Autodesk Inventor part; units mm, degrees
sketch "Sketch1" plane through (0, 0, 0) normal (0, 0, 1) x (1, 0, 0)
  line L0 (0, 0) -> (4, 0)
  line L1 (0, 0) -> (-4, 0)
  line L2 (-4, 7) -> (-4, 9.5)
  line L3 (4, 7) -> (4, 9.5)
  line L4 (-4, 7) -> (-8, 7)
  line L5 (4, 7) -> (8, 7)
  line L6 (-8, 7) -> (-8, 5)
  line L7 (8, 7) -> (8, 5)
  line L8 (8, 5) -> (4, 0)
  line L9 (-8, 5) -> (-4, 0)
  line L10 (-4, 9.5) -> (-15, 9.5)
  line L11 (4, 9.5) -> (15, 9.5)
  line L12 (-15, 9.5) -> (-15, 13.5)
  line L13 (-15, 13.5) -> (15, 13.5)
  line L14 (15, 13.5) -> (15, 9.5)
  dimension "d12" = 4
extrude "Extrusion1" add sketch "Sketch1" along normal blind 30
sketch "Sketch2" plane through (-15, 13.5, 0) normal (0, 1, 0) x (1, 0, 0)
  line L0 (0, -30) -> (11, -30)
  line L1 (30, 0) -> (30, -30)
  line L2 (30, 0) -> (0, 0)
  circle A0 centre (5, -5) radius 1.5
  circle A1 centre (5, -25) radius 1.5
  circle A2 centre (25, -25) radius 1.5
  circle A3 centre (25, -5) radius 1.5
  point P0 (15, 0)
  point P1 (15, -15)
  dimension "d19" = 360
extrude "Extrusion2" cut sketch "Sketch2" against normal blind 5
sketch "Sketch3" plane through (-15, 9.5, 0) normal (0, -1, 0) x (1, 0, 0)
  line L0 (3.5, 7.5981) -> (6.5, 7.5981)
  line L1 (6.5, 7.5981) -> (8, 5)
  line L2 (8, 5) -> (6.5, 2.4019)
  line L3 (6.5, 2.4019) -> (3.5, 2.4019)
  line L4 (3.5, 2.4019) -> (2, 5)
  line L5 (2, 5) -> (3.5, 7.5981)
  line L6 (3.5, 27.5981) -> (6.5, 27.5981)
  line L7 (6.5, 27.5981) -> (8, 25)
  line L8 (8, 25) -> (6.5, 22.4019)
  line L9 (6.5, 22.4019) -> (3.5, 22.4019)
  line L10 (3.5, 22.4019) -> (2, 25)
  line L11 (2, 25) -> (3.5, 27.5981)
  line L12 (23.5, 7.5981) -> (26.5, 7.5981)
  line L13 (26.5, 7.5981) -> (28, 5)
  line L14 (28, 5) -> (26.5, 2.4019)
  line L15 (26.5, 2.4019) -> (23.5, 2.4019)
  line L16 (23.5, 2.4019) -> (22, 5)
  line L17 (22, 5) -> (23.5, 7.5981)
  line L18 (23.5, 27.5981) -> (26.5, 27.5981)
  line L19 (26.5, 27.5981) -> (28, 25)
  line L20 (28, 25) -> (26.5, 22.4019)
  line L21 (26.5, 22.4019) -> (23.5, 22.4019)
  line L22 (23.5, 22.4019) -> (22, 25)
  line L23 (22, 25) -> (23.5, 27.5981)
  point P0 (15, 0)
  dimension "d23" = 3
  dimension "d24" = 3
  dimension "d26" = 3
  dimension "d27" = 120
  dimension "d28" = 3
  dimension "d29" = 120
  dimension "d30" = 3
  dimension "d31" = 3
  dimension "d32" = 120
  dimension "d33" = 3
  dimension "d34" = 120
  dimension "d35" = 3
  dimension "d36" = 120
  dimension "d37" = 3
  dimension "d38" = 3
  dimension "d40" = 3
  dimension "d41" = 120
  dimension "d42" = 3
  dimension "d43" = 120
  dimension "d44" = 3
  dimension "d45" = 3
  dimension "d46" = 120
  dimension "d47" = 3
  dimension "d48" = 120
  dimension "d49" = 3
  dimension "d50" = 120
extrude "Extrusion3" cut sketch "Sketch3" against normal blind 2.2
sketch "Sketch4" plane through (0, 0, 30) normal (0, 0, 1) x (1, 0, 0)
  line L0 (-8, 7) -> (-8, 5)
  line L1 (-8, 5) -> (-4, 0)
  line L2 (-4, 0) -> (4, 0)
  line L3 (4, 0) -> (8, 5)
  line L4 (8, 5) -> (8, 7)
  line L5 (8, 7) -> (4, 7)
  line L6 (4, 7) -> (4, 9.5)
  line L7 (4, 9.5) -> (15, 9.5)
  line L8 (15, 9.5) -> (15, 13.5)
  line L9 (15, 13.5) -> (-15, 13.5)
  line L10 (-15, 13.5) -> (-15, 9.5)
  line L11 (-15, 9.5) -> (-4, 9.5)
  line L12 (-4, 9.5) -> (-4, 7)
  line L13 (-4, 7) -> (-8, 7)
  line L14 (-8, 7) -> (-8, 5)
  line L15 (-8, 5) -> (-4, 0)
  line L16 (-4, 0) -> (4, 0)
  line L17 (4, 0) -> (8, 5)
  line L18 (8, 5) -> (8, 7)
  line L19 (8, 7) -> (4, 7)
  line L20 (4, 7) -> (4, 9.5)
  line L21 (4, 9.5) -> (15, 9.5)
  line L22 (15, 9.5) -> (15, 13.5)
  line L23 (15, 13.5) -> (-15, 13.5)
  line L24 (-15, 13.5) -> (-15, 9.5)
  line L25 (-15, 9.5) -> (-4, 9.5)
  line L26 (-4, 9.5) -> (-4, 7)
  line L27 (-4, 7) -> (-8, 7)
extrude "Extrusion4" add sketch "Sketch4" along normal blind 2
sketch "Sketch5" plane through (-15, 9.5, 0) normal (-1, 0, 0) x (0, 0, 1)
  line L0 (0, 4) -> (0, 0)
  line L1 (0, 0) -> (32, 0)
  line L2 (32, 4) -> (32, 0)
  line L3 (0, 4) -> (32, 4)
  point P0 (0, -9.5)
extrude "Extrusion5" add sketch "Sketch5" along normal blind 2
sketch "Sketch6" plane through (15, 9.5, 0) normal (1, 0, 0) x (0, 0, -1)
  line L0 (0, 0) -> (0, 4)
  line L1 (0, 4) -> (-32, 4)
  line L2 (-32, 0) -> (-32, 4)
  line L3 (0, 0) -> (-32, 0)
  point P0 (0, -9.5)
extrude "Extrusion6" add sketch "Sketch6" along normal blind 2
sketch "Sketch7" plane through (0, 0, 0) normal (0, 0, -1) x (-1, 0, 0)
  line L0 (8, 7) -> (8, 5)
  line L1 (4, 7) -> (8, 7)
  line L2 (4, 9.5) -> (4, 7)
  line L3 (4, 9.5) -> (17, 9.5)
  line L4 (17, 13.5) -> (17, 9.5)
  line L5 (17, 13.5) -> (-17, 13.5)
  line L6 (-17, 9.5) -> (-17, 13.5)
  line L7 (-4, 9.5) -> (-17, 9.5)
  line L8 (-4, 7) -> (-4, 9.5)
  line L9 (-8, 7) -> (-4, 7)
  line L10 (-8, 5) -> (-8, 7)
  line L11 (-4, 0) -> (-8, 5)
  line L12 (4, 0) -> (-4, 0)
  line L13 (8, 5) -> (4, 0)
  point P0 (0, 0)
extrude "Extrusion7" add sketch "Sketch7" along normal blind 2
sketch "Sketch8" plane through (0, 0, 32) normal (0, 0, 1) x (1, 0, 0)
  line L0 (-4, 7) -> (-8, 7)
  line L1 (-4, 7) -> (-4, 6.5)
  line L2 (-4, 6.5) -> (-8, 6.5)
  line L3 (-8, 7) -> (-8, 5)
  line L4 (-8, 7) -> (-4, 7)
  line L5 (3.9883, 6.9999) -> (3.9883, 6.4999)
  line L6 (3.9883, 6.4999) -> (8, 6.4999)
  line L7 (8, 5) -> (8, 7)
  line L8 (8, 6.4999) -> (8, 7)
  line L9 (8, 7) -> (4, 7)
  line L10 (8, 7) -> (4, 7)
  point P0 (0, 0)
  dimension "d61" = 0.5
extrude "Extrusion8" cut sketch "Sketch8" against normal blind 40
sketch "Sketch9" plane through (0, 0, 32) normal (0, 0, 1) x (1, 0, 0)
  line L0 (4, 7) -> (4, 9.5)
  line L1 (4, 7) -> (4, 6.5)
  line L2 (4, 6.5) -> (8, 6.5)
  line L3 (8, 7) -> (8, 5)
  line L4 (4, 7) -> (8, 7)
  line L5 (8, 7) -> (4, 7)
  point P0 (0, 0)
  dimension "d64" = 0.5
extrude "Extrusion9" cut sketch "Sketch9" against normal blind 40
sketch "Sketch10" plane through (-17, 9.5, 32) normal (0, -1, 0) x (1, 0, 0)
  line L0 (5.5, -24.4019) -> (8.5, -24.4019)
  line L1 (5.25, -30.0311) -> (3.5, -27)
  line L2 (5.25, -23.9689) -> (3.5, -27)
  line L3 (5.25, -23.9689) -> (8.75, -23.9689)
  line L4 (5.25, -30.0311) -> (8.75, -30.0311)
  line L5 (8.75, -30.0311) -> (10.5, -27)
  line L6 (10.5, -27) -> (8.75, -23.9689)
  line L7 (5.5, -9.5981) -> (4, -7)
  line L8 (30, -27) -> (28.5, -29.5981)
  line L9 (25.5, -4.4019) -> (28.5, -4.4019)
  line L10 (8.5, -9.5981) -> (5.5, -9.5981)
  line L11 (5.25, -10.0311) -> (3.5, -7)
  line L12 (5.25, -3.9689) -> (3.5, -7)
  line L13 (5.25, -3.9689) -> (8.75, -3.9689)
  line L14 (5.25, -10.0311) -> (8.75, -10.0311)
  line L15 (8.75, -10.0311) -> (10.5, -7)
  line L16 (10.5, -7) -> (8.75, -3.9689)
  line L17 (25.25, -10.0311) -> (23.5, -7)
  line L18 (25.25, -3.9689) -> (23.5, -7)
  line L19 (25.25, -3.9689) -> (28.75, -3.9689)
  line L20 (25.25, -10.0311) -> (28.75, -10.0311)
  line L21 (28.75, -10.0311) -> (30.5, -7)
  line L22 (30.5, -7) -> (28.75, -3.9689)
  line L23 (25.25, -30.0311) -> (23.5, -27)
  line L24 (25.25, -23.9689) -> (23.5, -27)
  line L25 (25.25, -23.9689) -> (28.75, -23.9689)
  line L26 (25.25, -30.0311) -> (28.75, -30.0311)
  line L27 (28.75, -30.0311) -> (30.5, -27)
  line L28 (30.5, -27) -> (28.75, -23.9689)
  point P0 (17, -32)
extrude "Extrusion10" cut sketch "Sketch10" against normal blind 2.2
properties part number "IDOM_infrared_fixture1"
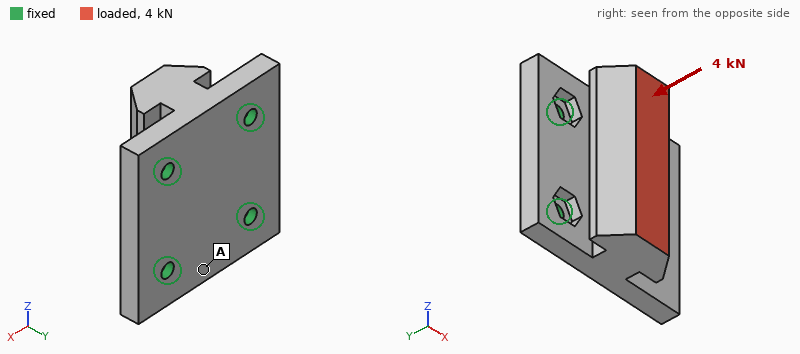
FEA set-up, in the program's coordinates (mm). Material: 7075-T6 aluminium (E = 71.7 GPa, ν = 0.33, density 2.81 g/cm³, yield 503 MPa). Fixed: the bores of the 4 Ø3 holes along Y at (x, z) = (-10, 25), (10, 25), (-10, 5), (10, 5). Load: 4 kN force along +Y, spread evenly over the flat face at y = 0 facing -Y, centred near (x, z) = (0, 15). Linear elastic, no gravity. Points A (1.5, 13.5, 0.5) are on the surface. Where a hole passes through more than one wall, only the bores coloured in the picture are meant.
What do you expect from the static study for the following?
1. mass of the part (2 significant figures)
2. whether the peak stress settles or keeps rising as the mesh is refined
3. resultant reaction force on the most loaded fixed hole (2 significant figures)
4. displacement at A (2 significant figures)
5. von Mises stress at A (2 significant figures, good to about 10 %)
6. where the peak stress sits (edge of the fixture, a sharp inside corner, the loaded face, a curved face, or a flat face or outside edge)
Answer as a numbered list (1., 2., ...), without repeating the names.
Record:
1. 22 g
2. keeps rising
3. 1.3 kN
4. 21 µm
5. 43 MPa
6. edge of the fixture
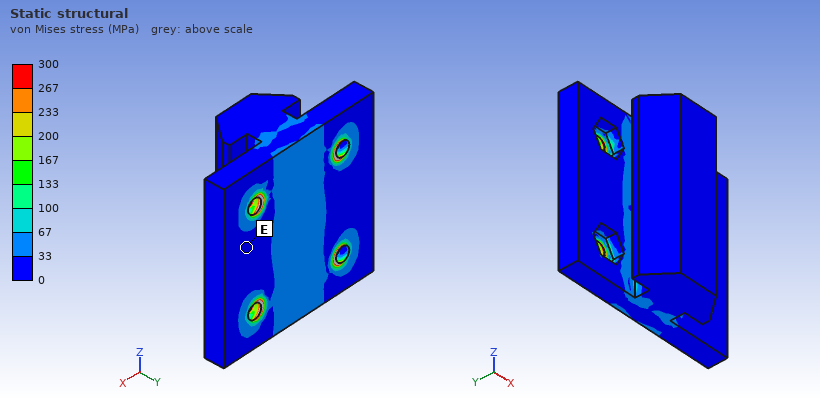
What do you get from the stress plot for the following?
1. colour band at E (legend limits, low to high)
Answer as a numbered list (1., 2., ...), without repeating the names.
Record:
1. 0 to 33 MPa
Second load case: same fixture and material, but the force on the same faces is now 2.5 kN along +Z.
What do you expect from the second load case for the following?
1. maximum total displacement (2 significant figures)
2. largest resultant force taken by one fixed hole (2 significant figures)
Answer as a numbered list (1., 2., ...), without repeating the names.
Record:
1. 39 µm
2. 1.1 kN
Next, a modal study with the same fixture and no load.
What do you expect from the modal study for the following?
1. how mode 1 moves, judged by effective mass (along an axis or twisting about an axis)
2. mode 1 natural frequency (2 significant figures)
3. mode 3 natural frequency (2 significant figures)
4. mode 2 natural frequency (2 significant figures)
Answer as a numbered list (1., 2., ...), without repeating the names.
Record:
1. along Z
2. 15 kHz
3. 18 kHz
4. 18 kHz
